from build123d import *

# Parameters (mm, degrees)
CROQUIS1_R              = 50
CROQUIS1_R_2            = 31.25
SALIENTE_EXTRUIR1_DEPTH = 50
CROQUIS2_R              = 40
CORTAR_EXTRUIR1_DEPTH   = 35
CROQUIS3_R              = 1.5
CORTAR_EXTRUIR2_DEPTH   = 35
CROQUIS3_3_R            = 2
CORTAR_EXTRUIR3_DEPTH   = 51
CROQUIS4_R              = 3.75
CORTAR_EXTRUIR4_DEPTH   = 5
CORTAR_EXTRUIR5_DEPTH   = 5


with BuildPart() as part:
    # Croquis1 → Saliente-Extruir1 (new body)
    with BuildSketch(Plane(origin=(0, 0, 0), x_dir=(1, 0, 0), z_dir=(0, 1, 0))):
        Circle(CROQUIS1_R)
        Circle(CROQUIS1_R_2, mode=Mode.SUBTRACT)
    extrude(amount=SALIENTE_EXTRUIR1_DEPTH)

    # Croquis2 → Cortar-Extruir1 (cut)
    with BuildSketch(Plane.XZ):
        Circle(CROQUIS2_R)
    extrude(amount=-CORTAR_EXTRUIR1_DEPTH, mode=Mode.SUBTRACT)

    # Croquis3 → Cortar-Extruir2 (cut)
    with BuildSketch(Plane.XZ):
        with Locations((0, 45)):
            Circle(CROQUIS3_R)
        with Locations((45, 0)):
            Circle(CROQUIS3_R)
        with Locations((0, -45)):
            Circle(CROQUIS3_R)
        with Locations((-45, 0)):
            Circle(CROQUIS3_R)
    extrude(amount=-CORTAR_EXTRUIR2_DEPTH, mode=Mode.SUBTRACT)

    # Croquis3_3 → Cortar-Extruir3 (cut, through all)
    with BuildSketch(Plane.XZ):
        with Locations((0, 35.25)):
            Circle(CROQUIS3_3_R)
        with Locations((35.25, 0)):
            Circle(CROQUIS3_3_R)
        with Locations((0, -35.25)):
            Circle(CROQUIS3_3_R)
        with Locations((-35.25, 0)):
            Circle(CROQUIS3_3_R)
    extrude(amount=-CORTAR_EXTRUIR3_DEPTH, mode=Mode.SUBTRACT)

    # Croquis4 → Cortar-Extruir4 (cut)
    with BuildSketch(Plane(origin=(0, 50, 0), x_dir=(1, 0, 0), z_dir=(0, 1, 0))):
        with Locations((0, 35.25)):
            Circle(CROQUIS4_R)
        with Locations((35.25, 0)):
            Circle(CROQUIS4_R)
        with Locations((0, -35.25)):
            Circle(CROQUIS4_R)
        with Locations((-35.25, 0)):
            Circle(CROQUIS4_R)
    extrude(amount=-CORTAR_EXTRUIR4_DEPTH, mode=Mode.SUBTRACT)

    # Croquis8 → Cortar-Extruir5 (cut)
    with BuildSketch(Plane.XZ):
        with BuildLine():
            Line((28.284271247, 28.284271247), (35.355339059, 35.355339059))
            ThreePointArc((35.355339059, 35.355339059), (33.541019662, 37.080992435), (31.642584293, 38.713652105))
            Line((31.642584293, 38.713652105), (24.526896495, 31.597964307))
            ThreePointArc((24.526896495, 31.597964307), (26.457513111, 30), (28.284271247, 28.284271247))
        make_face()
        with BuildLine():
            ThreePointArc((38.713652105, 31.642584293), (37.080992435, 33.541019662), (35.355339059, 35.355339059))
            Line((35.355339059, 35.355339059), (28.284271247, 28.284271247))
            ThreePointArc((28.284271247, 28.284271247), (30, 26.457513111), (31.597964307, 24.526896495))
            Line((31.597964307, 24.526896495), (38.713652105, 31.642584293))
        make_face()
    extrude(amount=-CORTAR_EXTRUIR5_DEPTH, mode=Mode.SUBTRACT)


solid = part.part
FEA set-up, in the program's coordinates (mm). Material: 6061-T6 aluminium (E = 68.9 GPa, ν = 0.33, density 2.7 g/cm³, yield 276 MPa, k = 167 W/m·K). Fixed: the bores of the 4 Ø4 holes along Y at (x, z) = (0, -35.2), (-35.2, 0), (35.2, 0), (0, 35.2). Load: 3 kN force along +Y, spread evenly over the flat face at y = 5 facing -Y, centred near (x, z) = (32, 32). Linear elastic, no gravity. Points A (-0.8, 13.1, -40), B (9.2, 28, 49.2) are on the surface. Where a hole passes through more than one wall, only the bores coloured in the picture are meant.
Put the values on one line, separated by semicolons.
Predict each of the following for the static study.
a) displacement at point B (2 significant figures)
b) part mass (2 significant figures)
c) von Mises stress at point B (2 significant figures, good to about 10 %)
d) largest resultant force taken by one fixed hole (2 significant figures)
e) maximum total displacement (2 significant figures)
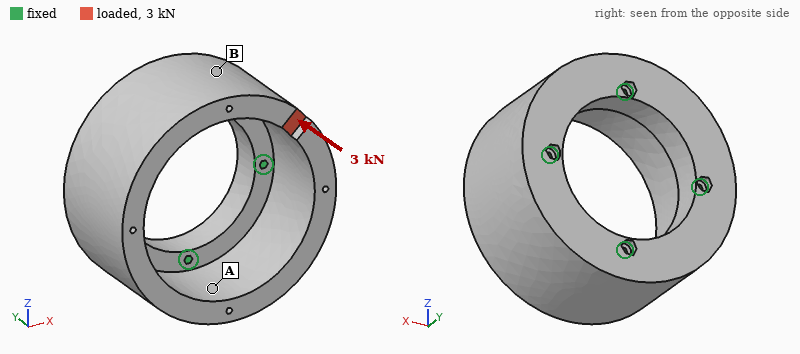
9.9 µm; 450 g; 10 MPa; 1.9 kN; 30 µm
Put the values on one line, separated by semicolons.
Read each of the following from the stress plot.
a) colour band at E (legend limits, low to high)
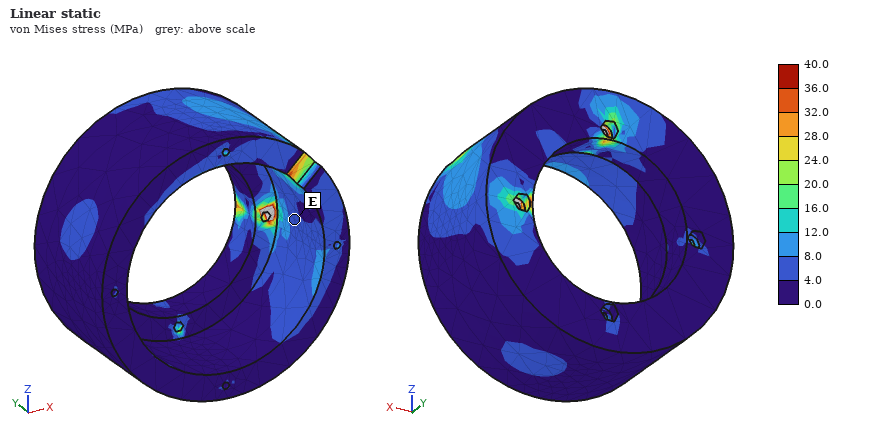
4.0 to 8.0 MPa
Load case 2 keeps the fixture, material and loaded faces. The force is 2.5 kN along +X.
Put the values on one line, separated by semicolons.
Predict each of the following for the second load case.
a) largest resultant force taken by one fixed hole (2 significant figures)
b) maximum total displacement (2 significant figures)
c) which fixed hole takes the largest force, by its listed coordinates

2.0 kN; 54 µm; (0, 35.2)
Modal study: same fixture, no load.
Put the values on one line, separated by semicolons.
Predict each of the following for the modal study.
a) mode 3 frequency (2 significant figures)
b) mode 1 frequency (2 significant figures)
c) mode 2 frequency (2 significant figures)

6100 Hz; 4800 Hz; 6100 Hz
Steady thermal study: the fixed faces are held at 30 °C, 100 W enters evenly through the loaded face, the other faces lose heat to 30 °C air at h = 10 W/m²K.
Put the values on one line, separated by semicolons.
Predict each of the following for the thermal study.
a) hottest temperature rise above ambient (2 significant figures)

65 K
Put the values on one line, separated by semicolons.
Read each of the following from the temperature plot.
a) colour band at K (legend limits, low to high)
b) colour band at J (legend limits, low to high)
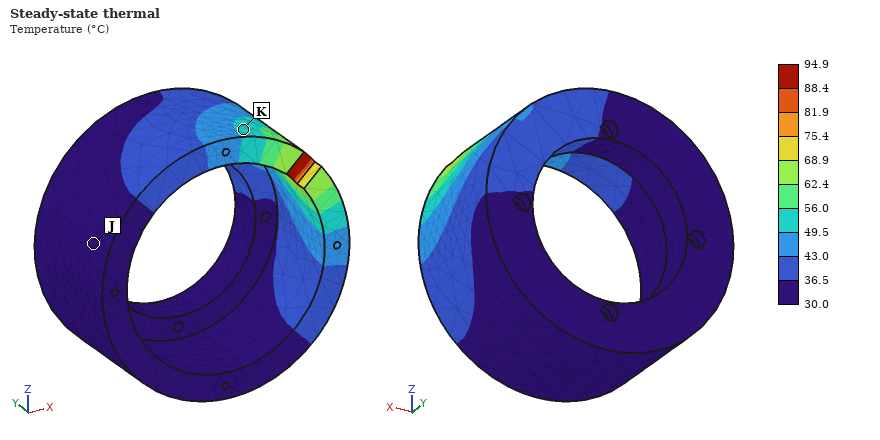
49.5 to 56.0 °C; 30.0 to 36.5 °C
